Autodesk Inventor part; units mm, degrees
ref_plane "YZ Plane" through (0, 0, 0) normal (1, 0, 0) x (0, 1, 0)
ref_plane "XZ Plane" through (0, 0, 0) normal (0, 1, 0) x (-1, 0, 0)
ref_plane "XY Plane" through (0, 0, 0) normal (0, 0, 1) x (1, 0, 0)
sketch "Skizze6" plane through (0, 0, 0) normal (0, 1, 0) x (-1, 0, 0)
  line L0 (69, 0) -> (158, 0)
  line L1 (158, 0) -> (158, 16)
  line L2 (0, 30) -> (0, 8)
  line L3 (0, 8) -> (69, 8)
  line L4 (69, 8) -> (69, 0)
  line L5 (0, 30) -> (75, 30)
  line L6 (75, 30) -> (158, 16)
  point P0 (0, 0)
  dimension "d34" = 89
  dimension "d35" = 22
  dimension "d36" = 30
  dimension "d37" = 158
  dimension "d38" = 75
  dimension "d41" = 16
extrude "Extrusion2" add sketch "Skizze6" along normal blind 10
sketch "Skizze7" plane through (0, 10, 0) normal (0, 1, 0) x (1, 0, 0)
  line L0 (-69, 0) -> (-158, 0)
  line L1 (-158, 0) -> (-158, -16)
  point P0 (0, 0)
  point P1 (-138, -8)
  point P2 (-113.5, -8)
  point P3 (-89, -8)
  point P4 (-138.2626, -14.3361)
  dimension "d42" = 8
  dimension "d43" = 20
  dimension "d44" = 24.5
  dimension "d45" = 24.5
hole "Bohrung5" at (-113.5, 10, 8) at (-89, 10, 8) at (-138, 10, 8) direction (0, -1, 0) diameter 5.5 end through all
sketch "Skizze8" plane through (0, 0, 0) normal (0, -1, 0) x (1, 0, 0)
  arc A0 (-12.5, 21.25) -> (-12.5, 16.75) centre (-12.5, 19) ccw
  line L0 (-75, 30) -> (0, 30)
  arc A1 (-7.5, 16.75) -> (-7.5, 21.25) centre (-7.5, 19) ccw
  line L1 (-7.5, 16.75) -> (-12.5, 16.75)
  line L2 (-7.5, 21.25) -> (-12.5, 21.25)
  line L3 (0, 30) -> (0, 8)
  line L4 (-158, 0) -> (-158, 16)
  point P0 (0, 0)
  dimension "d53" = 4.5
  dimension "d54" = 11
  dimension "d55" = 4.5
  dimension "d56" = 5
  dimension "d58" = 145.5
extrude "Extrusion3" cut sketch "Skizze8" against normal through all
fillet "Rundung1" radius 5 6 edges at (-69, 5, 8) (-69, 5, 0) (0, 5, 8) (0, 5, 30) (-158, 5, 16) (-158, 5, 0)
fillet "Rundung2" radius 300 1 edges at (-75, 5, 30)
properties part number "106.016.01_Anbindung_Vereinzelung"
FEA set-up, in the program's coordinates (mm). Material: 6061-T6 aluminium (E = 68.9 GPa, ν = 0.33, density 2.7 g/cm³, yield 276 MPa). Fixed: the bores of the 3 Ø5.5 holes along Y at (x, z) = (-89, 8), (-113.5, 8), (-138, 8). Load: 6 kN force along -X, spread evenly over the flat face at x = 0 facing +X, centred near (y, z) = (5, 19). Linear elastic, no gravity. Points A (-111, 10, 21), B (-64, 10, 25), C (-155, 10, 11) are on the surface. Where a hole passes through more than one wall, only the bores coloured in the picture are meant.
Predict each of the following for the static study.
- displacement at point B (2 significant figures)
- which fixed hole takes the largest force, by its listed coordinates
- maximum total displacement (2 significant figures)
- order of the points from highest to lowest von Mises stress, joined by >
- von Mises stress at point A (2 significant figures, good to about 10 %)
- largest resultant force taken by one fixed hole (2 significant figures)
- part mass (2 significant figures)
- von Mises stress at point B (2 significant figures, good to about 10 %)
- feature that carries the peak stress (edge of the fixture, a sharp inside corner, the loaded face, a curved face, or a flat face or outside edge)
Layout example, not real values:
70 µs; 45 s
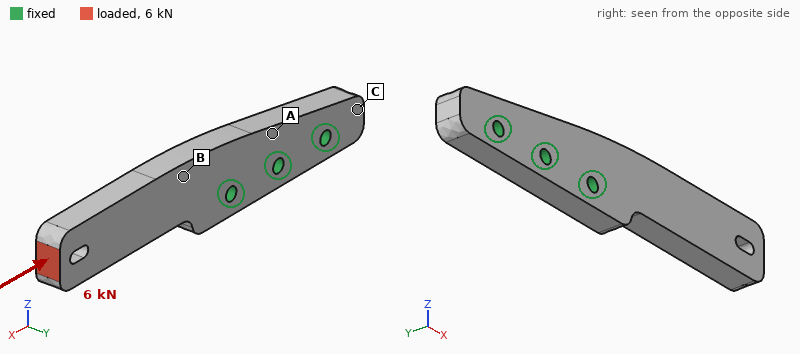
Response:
0.036 mm; (-89, 8); 0.11 mm; B > A > C; 17 MPa; 4.1 kN; 93 g; 29 MPa; a curved face
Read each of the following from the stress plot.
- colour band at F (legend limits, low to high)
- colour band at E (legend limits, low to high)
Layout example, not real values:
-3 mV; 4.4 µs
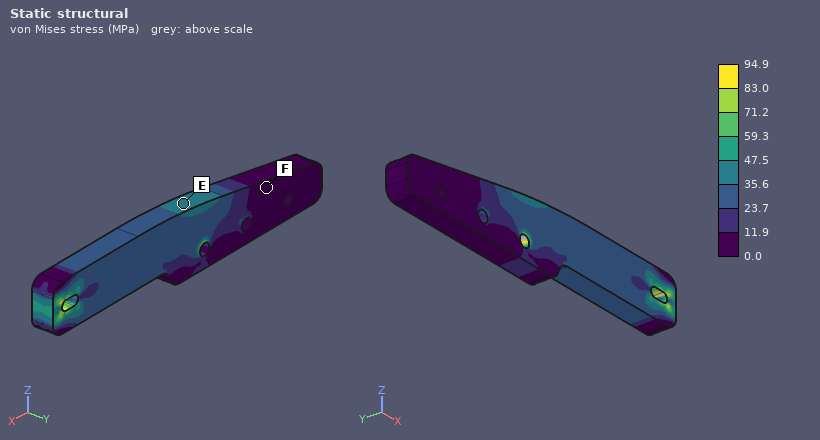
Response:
0.0 to 11.9 MPa; 35.6 to 47.5 MPa
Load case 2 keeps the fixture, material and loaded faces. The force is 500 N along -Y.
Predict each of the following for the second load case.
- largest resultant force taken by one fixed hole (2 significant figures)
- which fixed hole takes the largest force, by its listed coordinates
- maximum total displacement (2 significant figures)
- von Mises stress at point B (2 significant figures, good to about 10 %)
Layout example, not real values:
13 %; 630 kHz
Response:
1.1 kN; (-89, 8); 0.92 mm; 82 MPa
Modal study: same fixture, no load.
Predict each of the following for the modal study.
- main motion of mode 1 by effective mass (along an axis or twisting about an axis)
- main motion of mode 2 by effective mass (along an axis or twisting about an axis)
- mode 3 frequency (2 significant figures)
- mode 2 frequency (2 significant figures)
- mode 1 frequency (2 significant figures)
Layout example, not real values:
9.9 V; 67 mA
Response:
along Y; along Z; 5500 Hz; 2300 Hz; 1100 Hz
